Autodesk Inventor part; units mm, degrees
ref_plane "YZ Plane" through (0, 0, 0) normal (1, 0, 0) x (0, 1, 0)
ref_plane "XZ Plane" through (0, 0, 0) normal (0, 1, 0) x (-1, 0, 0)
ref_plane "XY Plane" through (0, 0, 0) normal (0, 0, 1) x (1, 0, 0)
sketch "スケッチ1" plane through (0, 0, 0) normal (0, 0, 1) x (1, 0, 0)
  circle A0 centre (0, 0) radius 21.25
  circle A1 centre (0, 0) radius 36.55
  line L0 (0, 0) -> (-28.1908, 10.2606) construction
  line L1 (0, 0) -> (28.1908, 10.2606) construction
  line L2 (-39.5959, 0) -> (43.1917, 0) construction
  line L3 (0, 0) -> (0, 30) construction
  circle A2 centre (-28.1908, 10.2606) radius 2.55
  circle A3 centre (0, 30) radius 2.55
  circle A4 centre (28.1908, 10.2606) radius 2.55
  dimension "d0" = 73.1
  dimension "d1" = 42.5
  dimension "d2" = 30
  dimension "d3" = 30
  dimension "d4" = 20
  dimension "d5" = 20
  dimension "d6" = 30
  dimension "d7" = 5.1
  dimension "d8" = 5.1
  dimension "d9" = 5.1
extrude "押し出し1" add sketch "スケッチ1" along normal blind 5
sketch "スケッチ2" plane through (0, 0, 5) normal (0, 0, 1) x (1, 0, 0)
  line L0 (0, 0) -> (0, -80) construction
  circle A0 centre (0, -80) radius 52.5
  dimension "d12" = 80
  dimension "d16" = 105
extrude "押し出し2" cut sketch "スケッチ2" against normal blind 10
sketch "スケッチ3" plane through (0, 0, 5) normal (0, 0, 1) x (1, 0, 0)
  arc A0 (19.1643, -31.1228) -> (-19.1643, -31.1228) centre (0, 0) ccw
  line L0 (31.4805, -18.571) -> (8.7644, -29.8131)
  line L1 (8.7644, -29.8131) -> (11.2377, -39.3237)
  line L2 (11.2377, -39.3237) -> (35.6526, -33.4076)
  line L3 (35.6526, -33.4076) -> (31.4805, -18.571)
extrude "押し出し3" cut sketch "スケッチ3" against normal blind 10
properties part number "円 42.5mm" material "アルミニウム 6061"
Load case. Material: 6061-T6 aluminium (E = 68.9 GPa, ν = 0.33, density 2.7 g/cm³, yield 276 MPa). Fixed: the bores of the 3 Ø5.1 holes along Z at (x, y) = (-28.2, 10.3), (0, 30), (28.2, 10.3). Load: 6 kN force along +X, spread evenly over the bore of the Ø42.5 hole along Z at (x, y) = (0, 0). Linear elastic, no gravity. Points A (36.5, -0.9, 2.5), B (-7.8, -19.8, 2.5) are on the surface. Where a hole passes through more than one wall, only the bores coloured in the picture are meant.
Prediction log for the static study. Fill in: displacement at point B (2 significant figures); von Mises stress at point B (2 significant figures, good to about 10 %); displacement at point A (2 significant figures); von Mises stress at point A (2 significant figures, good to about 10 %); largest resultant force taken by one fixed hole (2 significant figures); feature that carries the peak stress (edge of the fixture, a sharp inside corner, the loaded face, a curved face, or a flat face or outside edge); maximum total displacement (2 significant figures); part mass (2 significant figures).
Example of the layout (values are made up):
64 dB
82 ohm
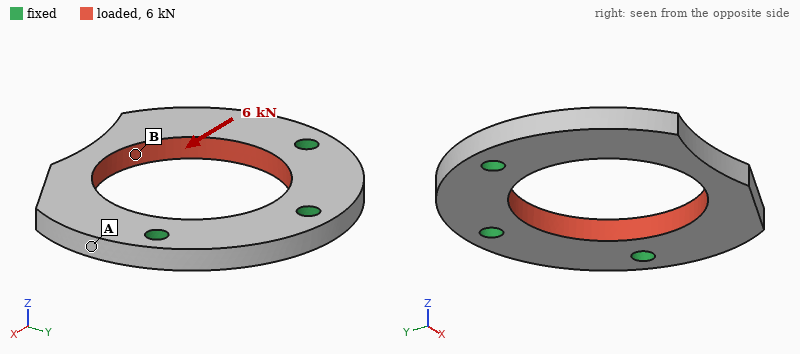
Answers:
94 µm
110 MPa
39 µm
32 MPa
2.8 kN
edge of the fixture
98 µm
32 g
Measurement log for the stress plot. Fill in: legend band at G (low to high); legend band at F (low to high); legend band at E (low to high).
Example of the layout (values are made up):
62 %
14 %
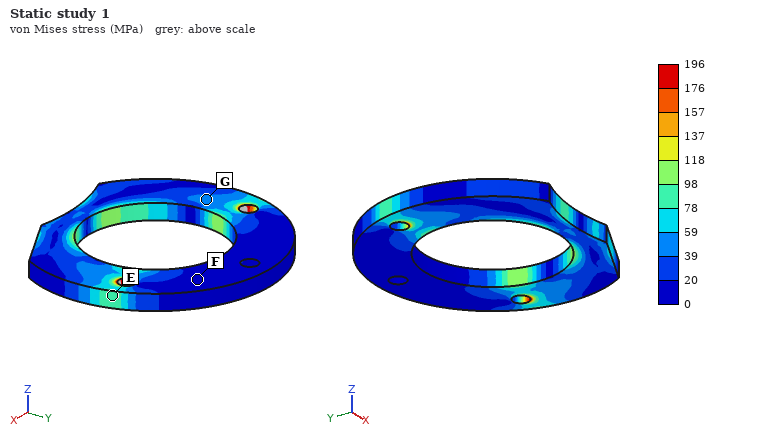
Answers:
39 to 59 MPa
0 to 20 MPa
78 to 98 MPa
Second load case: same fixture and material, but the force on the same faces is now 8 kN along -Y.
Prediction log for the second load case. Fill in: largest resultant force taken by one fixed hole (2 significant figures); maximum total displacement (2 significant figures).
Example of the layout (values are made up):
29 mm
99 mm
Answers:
3.3 kN
51 µm
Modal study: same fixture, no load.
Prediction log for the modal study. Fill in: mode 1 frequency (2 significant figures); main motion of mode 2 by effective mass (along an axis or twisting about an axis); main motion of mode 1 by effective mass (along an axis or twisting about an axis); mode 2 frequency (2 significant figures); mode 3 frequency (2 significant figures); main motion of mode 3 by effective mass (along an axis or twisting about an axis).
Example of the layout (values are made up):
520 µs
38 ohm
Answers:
2300 Hz
twisting about Y
along Z
4700 Hz
8100 Hz
along X
